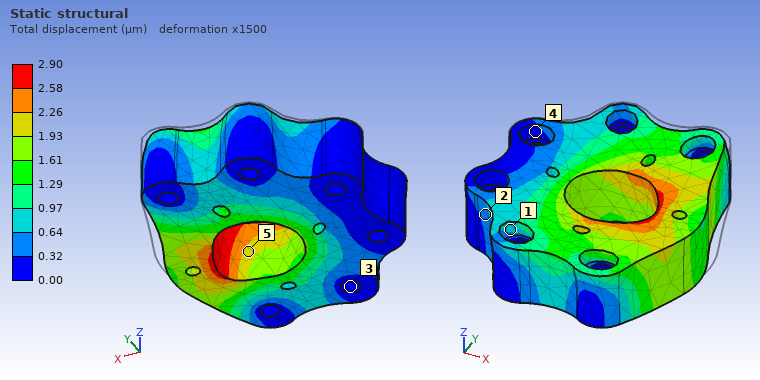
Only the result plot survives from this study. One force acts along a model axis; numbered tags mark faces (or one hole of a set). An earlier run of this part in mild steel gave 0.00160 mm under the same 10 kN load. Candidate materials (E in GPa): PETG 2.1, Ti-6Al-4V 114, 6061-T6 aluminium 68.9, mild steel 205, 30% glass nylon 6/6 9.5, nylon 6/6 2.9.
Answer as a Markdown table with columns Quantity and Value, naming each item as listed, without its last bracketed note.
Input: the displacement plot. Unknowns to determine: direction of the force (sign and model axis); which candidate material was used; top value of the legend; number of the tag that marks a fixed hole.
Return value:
| Quantity | Value |
|---|---|
| direction of the force | -Y |
| which candidate material was used | Ti-6Al-4V |
| top value of the legend | 2.90 µm |
| number of the tag that marks a fixed hole | 3 |
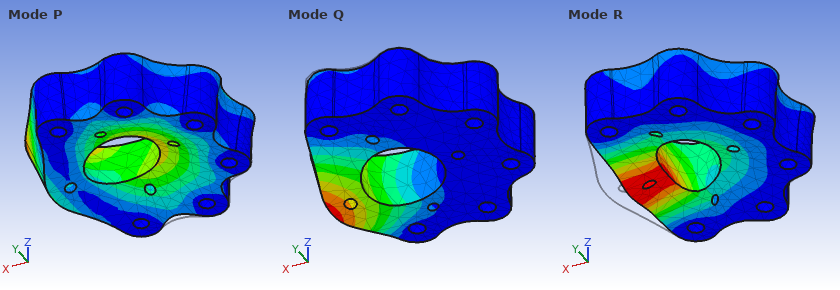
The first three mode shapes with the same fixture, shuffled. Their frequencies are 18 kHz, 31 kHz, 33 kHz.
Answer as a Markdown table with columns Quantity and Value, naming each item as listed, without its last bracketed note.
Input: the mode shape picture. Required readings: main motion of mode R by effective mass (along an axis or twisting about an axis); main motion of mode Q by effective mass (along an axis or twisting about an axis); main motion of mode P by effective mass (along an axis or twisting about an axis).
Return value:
| Quantity | Value |
|---|---|
| main motion of mode R by effective mass | along X |
| main motion of mode Q by effective mass | along Z |
| main motion of mode P by effective mass | along Z |
